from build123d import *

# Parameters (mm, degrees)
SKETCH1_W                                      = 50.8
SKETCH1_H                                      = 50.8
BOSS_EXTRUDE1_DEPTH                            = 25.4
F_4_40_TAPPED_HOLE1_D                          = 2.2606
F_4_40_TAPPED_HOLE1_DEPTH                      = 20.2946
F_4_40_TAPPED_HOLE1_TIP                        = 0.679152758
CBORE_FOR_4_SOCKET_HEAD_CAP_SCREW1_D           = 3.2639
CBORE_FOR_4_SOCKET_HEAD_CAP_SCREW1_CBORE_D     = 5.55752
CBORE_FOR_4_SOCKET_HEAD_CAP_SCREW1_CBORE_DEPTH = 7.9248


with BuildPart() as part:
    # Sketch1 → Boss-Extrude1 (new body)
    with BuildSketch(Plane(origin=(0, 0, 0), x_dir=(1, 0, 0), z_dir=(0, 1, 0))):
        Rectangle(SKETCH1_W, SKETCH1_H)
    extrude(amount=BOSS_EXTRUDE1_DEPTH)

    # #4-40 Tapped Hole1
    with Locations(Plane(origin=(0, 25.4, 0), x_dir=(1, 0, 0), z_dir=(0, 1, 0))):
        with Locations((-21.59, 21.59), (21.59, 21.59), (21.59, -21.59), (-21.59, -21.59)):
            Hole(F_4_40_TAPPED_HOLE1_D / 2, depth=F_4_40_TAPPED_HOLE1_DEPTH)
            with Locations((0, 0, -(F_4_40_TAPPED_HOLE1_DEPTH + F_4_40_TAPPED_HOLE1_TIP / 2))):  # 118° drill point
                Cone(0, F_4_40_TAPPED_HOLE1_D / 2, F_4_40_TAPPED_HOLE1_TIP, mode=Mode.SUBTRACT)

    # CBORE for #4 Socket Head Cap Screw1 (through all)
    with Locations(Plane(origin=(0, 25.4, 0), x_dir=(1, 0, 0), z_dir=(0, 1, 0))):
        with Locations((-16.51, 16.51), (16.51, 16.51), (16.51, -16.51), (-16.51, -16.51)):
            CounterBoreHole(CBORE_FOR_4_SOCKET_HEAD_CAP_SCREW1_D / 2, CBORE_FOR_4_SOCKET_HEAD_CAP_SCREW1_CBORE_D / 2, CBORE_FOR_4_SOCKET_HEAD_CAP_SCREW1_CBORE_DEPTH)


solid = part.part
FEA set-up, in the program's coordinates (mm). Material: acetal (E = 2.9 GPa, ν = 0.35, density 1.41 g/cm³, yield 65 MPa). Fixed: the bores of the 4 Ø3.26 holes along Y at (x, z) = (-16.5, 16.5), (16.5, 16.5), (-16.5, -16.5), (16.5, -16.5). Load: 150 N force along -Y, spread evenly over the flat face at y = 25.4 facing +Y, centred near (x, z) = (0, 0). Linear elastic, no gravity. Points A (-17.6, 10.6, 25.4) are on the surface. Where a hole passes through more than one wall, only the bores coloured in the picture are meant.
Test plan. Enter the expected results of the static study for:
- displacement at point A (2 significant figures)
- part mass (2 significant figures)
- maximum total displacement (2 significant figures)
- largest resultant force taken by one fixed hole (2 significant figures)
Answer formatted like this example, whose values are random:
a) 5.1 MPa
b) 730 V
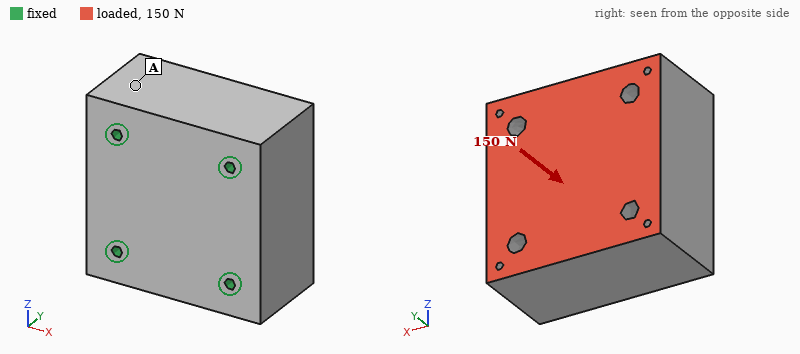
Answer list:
a) 0.38 µm
b) 90 g
c) 1.0 µm
d) 38 N
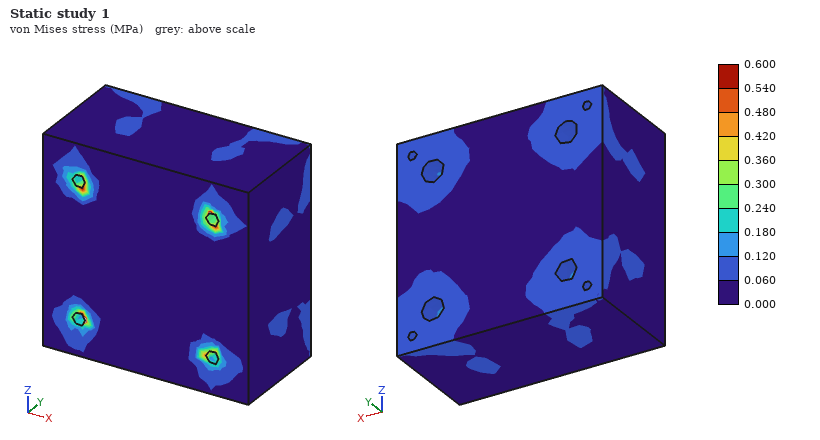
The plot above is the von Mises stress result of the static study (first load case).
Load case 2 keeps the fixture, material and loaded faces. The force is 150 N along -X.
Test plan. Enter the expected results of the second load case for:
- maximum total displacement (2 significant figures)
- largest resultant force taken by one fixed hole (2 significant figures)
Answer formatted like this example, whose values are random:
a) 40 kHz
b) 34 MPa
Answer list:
a) 2.7 µm
b) 47 N
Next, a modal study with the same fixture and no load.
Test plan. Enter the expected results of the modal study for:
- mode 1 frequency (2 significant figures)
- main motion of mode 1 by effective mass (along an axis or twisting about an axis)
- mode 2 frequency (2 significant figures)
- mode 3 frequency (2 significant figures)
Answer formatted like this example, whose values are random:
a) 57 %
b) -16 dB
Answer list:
a) 7700 Hz
b) along Y
c) 8200 Hz
d) 8200 Hz
